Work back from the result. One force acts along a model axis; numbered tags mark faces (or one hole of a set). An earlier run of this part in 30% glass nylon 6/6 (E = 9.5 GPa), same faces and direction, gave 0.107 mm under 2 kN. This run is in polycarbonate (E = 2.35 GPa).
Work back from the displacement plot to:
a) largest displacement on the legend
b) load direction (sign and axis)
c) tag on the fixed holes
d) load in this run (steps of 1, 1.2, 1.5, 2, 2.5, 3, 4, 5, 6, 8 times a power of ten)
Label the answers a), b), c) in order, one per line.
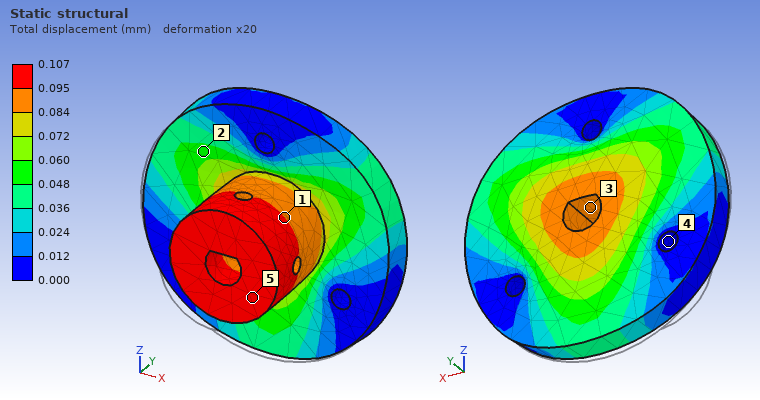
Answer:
a) 0.107 mm
b) +Y
c) 4
d) 500 N
